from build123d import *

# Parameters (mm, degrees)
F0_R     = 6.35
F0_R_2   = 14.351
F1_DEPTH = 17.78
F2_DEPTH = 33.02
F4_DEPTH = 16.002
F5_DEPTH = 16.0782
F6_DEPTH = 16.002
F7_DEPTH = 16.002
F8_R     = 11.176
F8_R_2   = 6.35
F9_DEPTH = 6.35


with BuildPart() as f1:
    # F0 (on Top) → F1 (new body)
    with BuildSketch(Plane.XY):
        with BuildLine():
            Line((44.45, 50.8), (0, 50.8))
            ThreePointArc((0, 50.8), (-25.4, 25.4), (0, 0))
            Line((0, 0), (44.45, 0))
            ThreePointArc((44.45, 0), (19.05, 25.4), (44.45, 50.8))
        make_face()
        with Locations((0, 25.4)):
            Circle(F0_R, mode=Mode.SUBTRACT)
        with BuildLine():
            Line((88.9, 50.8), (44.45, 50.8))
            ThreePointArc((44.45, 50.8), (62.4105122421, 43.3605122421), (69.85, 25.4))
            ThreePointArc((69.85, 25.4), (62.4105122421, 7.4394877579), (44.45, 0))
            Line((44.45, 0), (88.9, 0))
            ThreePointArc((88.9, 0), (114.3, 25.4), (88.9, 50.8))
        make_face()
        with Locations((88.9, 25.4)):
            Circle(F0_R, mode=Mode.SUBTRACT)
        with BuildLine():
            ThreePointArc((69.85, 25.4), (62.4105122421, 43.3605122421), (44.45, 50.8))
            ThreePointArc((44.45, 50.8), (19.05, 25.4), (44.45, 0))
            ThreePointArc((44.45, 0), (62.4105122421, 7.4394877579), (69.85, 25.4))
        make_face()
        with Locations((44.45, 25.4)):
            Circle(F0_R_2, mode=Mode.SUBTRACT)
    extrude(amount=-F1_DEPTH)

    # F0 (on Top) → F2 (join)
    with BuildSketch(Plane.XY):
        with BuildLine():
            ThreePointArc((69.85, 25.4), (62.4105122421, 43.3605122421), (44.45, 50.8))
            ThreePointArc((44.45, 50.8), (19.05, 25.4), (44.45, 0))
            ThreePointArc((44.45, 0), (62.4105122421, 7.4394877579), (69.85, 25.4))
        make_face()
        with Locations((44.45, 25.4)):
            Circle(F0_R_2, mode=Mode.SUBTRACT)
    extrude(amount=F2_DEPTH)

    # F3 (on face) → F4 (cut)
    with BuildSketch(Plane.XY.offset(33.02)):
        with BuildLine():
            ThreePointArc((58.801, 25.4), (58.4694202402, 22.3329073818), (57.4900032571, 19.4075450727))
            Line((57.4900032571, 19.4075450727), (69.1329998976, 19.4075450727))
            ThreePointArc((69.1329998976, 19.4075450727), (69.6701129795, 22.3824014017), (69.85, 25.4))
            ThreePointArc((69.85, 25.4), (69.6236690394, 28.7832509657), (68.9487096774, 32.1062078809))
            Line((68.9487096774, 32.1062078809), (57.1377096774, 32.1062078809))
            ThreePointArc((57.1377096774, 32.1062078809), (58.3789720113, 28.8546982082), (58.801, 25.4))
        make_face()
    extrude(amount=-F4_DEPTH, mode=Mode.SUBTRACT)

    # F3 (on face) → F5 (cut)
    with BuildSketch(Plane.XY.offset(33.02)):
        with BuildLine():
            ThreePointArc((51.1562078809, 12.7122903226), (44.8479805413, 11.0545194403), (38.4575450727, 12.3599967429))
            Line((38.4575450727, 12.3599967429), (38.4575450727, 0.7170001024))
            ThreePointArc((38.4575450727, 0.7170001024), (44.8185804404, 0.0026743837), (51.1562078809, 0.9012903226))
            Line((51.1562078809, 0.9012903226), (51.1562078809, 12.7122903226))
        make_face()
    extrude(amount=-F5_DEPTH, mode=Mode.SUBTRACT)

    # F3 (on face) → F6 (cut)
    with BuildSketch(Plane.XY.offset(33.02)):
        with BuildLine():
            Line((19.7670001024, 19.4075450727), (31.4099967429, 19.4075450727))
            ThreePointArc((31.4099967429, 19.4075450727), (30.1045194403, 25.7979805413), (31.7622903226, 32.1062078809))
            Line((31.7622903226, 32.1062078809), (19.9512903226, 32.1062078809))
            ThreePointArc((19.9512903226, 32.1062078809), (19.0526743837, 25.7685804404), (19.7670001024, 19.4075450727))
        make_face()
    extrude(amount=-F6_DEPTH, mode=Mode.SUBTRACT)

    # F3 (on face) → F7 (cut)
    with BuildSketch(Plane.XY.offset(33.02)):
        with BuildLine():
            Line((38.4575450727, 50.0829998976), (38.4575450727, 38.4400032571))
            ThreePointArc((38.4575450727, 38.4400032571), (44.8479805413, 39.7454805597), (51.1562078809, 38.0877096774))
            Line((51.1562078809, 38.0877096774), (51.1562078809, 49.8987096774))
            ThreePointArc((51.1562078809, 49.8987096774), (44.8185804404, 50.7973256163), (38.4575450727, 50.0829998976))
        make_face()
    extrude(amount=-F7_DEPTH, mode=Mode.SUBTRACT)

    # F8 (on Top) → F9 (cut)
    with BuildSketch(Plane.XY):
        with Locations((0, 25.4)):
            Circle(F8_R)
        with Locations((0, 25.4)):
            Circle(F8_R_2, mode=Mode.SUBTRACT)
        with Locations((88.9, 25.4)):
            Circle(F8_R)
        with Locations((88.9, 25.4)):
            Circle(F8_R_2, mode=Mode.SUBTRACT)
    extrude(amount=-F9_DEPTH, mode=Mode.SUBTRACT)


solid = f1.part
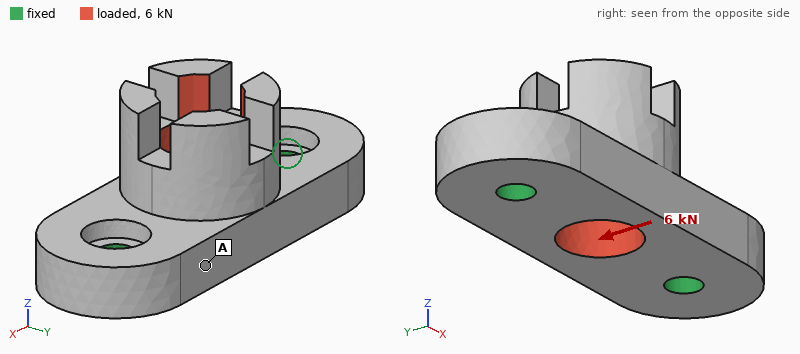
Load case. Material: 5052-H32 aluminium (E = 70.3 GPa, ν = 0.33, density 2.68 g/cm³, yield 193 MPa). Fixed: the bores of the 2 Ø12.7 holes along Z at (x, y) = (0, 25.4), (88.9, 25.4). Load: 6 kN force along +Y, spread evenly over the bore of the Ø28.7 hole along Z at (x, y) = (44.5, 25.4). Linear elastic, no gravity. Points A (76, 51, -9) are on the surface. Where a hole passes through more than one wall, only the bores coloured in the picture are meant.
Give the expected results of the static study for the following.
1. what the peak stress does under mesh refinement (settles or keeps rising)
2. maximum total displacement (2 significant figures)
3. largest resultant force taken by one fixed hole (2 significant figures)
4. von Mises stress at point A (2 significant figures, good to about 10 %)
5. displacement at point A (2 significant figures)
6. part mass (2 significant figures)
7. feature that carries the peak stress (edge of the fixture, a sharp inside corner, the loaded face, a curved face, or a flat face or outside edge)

keeps rising
56 µm
3.0 kN
11 MPa
17 µm
360 g
edge of the fixture
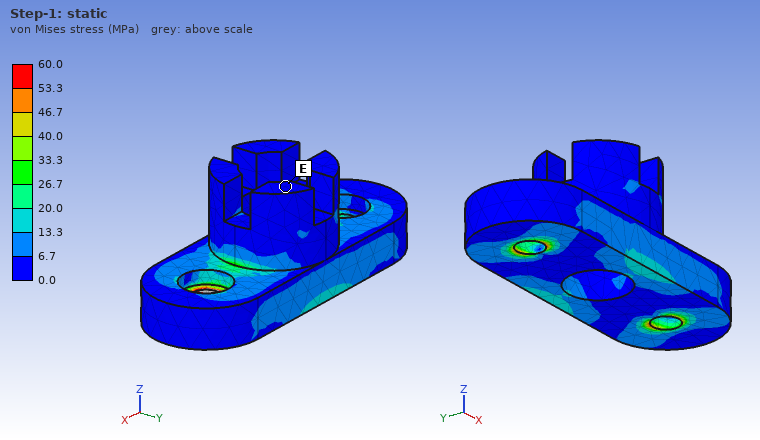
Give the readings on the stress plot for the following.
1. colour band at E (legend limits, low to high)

0.0 to 6.7 MPa
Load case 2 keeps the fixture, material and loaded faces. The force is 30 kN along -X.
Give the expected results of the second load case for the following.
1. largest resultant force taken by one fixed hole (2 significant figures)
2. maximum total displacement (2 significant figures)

16 kN
67 µm
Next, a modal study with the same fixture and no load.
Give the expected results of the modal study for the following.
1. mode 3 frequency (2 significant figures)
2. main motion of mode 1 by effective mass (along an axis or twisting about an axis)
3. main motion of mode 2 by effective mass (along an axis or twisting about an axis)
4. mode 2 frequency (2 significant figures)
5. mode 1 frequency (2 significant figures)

9600 Hz
along Y
along Z
7200 Hz
4300 Hz
